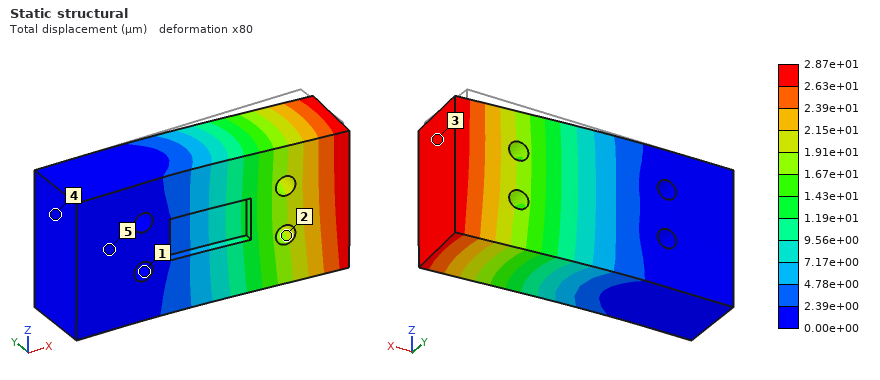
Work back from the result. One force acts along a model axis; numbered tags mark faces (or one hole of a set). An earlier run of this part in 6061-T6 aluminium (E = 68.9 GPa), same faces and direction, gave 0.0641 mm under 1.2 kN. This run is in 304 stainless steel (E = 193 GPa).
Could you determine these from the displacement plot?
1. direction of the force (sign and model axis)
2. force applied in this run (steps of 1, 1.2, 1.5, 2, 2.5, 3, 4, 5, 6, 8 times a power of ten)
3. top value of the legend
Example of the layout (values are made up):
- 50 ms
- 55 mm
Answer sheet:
- -Y
- 1.5 kN
- 2.87e+01 µm
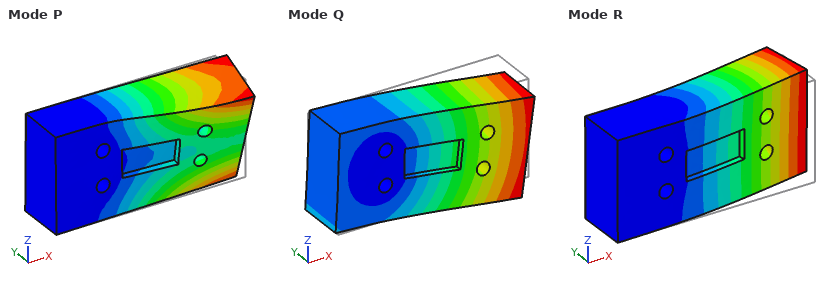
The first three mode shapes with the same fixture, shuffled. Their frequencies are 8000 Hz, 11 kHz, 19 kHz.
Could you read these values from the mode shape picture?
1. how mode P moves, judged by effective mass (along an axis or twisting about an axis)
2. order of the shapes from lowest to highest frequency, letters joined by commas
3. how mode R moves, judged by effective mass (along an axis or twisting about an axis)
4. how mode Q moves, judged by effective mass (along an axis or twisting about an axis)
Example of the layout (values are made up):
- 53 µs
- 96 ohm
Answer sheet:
- twisting about X
- R, Q, P
- along Y
- along Z
